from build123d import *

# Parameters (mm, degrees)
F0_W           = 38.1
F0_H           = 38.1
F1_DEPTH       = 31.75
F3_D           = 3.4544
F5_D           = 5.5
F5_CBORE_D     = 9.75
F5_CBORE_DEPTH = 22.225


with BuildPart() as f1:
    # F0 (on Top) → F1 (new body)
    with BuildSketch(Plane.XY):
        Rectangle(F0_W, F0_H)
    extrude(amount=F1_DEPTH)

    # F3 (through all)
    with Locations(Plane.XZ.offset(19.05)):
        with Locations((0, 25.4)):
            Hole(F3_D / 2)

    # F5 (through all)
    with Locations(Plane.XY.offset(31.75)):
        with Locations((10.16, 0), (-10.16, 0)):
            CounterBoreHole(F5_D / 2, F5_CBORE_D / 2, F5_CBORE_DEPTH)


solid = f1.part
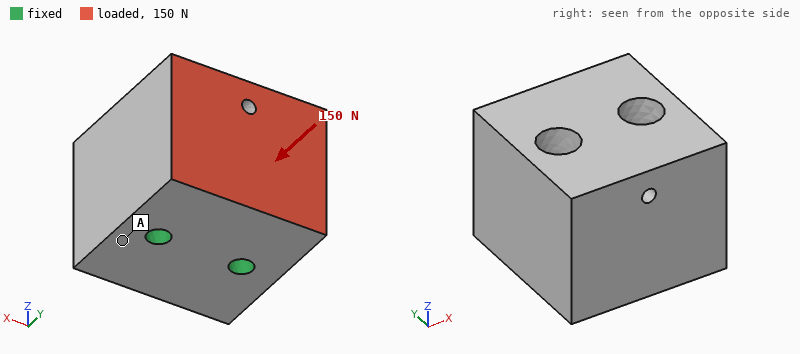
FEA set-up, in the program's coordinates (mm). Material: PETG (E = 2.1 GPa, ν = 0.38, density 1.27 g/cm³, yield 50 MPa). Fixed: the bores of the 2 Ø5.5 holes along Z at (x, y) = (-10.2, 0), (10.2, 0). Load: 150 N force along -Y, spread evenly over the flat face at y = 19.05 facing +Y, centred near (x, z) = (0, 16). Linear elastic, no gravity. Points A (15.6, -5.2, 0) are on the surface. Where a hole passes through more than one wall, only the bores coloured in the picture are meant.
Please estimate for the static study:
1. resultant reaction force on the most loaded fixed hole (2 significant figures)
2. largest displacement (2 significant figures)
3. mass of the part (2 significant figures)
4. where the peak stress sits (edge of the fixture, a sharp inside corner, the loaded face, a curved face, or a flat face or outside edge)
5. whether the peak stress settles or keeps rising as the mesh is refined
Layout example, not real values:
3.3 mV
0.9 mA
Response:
75 N
33 µm
53 g
edge of the fixture
keeps rising
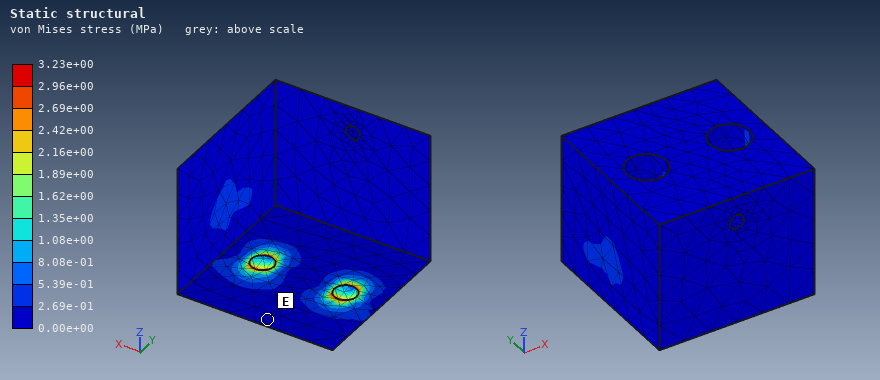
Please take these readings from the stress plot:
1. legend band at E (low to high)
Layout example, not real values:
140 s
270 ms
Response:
0.00e+00 to 2.69e-01 MPa
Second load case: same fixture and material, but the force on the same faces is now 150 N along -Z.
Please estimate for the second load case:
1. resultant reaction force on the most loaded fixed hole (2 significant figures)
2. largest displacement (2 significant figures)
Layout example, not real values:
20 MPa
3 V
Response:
76 N
56 µm
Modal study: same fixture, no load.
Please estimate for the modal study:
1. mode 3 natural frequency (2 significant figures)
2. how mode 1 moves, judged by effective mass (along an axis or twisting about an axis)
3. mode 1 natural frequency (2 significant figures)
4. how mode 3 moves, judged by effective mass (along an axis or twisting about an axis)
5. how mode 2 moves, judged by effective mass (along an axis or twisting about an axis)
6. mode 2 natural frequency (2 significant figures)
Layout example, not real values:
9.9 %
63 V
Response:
4000 Hz
along Y
1600 Hz
twisting about Z
along X
3000 Hz
